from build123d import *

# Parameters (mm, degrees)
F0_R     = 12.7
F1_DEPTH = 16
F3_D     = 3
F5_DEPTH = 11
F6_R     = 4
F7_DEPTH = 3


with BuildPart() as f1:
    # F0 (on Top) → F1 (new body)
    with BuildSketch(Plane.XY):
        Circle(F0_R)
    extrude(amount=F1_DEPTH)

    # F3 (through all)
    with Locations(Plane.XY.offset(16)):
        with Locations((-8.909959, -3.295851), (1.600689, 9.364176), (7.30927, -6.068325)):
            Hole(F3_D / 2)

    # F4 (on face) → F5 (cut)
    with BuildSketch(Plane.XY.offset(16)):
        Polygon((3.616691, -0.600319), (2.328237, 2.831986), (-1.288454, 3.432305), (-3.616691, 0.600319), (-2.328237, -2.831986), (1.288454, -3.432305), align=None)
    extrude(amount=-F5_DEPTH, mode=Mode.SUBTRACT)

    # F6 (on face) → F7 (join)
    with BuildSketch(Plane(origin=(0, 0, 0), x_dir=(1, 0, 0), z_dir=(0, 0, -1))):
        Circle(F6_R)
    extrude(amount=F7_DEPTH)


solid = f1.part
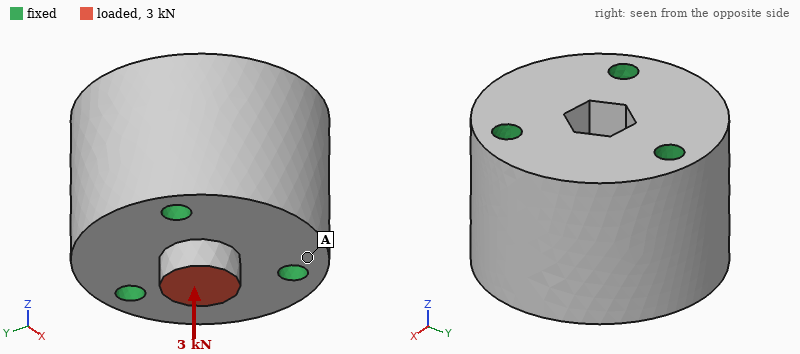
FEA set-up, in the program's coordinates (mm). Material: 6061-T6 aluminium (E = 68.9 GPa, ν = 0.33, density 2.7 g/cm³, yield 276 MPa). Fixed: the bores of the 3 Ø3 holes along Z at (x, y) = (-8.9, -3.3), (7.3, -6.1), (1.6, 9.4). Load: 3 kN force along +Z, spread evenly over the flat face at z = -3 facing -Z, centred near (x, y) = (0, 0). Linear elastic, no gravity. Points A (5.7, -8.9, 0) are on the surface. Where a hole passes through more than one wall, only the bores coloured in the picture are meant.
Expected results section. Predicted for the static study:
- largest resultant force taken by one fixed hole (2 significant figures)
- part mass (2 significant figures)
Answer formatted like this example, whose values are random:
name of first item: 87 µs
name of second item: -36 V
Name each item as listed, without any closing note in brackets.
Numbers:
largest resultant force taken by one fixed hole: 1.1 kN
part mass: 20 g
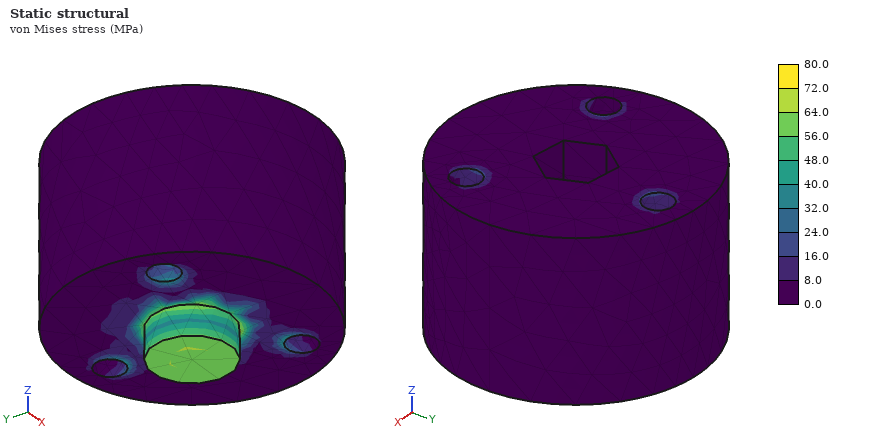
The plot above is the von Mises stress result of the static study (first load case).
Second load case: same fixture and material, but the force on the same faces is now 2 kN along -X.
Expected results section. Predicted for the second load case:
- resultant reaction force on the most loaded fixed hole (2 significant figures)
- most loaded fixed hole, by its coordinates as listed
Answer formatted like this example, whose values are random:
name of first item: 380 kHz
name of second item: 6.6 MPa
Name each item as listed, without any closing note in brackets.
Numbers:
resultant reaction force on the most loaded fixed hole: 1.1 kN
most loaded fixed hole, by its coordinates as listed: (-8.9, -3.3)
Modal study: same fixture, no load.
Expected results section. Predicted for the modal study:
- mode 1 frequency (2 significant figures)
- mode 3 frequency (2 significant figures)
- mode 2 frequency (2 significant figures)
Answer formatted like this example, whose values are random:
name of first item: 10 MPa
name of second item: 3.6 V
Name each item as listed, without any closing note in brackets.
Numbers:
mode 1 frequency: 70 kHz
mode 3 frequency: 72 kHz
mode 2 frequency: 70 kHz
